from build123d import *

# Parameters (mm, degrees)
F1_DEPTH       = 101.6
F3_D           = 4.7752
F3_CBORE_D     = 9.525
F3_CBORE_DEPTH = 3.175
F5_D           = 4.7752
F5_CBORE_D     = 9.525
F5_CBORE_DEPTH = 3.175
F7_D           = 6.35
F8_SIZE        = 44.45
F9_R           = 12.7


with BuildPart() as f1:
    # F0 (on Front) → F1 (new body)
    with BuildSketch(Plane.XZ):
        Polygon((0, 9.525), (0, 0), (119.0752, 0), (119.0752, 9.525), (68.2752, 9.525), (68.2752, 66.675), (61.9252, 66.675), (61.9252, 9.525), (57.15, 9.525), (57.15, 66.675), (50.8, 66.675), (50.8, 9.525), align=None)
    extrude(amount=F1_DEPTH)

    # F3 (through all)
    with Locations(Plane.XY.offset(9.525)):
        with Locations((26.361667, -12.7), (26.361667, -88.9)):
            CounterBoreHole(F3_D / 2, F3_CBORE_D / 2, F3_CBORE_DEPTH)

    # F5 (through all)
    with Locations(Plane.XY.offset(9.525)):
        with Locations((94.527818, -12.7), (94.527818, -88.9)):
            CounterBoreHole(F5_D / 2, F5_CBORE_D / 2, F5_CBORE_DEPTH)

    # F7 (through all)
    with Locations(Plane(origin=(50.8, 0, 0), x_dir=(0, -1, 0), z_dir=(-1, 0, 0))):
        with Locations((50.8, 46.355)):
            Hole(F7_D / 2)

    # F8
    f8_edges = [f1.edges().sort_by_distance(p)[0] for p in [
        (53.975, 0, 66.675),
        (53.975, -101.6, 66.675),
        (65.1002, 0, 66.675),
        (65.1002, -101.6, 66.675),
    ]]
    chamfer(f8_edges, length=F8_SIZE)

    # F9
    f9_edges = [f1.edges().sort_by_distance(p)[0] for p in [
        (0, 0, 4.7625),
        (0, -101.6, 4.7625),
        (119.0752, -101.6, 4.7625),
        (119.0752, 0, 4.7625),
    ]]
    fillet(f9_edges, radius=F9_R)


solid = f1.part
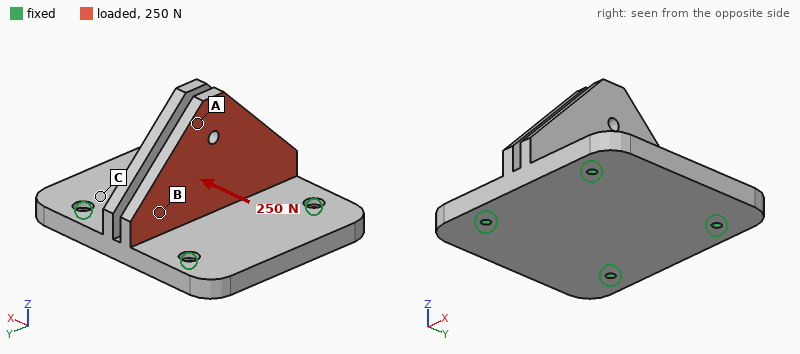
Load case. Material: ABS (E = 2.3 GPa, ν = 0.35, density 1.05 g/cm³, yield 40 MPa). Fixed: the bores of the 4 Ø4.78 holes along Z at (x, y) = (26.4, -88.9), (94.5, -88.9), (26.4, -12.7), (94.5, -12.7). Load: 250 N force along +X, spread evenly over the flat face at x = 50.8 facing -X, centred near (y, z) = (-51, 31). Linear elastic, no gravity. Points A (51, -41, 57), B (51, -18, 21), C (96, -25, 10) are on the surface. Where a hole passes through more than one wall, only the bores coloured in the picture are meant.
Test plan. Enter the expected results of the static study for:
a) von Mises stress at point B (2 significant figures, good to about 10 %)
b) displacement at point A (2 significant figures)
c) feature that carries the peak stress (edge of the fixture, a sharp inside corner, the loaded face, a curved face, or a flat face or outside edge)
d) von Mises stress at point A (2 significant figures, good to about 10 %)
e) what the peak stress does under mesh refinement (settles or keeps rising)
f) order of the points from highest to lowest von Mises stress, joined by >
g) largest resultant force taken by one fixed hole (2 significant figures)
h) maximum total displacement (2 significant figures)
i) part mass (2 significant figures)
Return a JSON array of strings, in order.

["4.3 MPa", "0.86 mm", "edge of the fixture", "1.3 MPa", "keeps rising", "B > A > C", "93 N", "1.1 mm", "170 g"]
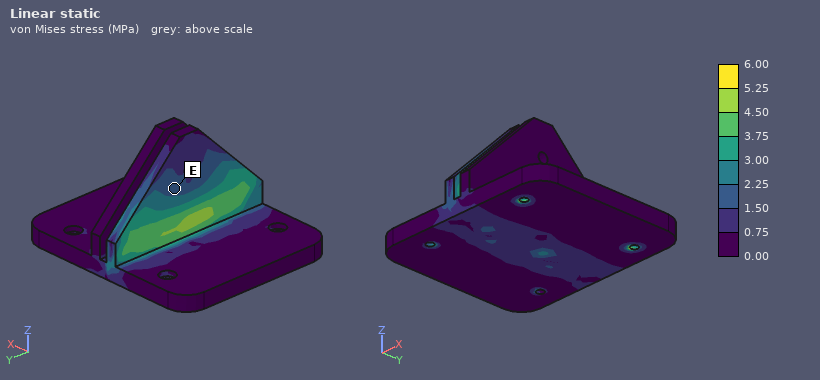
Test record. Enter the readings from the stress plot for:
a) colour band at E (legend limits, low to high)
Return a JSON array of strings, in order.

["1.50 to 2.25 MPa"]
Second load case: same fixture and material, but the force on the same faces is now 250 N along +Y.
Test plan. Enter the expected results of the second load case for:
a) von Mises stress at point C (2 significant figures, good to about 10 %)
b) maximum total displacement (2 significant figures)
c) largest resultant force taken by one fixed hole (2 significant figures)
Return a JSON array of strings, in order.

["0.38 MPa", "86 µm", "98 N"]
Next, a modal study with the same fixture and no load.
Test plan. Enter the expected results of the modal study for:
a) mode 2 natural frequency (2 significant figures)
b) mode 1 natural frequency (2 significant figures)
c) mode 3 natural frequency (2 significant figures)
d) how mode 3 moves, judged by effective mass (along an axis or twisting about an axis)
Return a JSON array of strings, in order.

["660 Hz", "650 Hz", "1200 Hz", "along Z"]
